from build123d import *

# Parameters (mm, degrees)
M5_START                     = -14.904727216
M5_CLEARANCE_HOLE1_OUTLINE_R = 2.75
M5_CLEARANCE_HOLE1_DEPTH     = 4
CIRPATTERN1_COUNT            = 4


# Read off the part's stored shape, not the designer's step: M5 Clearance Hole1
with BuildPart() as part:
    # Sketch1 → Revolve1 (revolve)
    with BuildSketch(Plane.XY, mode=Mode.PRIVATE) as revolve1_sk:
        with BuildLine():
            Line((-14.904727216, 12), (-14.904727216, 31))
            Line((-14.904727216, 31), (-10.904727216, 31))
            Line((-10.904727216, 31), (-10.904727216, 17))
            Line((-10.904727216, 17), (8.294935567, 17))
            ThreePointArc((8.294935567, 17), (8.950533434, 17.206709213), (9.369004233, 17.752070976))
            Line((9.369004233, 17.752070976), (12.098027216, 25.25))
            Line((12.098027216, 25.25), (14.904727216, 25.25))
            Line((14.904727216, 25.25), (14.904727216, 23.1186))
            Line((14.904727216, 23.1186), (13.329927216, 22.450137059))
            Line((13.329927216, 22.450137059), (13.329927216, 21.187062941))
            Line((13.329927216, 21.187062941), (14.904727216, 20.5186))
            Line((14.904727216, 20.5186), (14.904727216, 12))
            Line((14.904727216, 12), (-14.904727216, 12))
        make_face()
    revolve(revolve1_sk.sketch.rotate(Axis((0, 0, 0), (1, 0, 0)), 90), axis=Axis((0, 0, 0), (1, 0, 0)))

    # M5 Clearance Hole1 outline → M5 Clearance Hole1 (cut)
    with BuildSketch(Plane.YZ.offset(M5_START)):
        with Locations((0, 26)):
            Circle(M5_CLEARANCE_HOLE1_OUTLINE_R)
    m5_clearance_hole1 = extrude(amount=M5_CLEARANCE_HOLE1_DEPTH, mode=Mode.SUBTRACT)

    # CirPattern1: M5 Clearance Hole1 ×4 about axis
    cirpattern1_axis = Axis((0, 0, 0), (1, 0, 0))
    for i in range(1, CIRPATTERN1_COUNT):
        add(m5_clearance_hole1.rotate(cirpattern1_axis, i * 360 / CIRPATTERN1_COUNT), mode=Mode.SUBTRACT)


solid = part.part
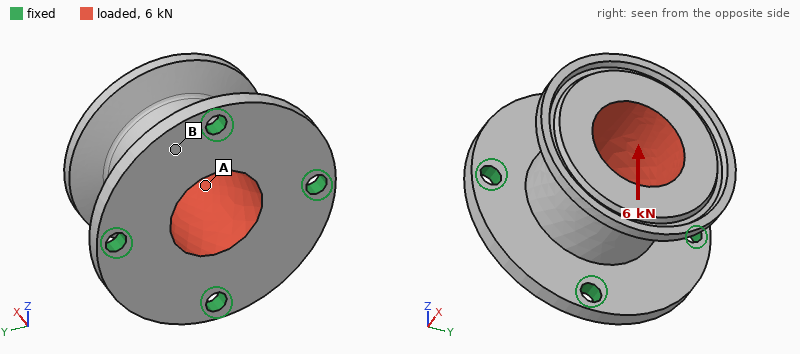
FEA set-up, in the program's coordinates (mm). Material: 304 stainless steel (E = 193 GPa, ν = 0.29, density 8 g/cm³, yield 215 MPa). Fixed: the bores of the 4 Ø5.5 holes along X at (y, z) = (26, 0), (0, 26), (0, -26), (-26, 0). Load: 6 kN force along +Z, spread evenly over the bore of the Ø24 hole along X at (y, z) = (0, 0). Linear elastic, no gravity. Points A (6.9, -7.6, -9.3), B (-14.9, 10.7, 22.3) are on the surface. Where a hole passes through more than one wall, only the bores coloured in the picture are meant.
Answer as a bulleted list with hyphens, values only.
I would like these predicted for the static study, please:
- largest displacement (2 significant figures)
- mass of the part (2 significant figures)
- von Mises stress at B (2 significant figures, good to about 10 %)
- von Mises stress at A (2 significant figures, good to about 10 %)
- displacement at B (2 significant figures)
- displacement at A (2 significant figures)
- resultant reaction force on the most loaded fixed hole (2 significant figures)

- 26 µm
- 210 g
- 25 MPa
- 14 MPa
- 5.1 µm
- 17 µm
- 2.5 kN
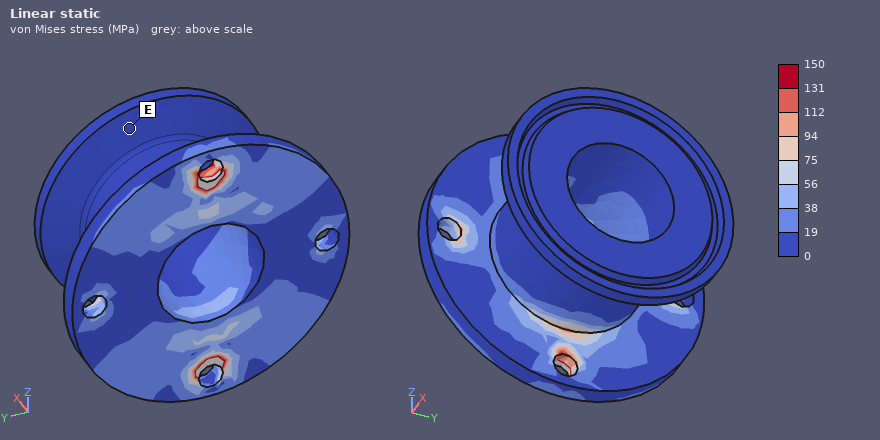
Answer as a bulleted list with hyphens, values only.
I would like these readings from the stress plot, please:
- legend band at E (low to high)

- 0 to 19 MPa
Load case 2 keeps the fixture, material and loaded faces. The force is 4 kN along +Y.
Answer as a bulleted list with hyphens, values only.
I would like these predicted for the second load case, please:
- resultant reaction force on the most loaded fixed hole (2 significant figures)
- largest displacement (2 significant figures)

- 1.7 kN
- 17 µm
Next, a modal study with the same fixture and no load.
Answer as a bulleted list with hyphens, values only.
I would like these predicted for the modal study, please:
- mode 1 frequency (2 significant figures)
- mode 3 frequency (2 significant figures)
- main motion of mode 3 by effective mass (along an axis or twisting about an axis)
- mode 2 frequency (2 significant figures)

- 6300 Hz
- 9200 Hz
- along X
- 6300 Hz
